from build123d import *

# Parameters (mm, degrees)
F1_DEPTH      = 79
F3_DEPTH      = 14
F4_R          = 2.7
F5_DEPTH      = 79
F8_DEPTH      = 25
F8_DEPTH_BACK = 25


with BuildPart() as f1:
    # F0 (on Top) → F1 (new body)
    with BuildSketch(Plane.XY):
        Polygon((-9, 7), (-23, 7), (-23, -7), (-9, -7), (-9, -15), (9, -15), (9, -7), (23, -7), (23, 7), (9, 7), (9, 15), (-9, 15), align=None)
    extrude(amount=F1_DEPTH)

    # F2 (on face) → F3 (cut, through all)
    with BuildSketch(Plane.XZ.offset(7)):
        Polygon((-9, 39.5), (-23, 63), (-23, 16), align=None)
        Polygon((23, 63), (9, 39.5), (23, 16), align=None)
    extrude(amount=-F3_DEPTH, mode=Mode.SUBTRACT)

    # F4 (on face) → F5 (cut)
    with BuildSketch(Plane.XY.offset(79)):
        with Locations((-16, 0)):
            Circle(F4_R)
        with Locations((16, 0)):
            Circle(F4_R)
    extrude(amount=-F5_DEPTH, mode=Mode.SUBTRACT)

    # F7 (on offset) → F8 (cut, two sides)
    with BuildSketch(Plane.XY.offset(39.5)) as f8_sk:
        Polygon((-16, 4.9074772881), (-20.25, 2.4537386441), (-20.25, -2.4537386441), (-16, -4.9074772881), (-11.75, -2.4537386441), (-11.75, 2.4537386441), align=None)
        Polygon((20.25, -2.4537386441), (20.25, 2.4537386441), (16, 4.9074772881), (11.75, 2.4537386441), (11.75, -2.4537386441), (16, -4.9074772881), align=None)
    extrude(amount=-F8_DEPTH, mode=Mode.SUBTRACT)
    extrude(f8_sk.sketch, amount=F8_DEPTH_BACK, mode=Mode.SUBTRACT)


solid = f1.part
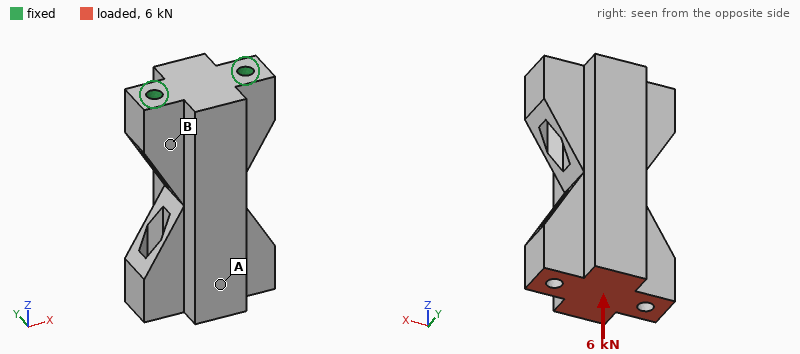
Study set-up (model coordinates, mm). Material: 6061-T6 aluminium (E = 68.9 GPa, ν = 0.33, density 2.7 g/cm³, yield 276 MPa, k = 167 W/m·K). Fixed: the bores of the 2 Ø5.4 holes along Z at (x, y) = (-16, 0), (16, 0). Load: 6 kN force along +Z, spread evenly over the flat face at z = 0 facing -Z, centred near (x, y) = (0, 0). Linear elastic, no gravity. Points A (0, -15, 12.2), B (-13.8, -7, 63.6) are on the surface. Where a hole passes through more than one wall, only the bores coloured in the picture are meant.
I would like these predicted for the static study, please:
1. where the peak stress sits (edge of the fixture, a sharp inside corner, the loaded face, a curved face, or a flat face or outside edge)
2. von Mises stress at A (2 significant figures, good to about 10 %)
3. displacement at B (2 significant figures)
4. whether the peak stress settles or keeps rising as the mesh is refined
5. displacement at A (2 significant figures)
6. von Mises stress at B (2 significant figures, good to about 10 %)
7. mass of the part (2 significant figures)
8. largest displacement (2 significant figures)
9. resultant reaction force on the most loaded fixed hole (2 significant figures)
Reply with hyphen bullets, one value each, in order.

- edge of the fixture
- 7.2 MPa
- 2.5 µm
- keeps rising
- 11 µm
- 16 MPa
- 160 g
- 14 µm
- 3.1 kN
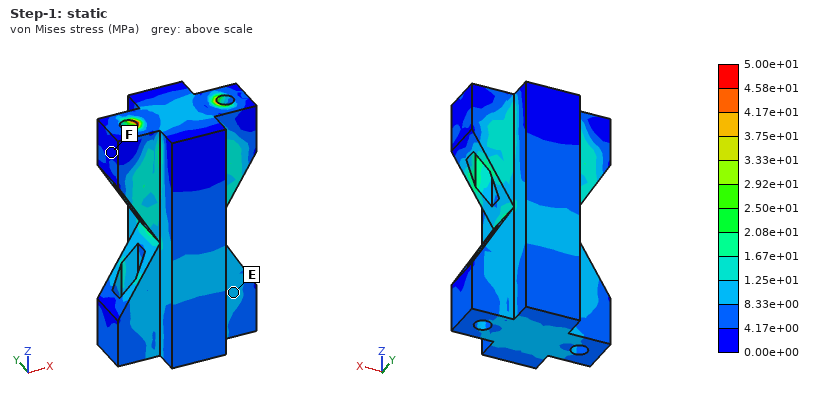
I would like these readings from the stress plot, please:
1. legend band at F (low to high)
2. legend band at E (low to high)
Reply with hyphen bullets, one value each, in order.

- 0.00e+00 to 4.17e+00 MPa
- 8.33e+00 to 1.25e+01 MPa
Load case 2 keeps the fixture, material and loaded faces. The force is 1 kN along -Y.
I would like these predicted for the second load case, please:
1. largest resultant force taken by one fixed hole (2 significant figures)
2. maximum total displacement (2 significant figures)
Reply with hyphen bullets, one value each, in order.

- 500 N
- 0.13 mm
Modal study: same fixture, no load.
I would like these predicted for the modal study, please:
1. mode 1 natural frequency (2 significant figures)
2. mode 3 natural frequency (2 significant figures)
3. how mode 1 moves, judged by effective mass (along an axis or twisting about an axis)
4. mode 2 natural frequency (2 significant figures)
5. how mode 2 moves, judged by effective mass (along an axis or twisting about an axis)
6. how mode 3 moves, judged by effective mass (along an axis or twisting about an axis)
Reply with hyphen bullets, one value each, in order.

- 2000 Hz
- 7400 Hz
- along Y
- 3300 Hz
- along X
- twisting about Z
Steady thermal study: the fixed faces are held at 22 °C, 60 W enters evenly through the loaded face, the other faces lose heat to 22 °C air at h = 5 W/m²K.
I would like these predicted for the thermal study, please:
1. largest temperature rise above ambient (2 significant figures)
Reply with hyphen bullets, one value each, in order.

- 40 K
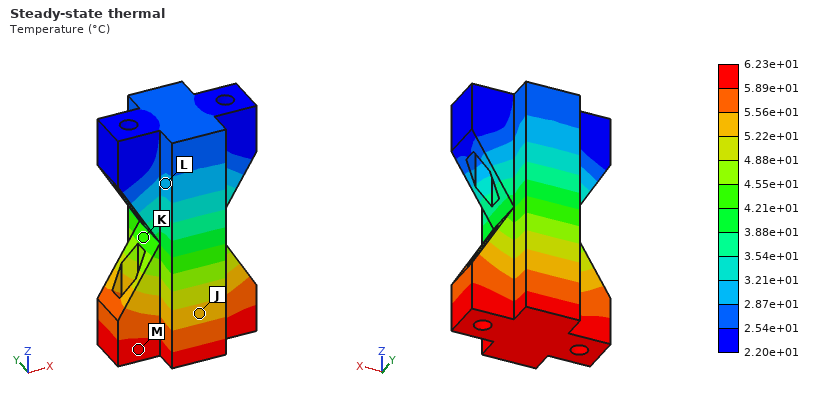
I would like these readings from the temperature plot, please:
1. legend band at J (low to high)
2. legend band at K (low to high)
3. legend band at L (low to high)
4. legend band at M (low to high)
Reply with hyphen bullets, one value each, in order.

- 5.22e+01 to 5.56e+01 °C
- 4.21e+01 to 4.55e+01 °C
- 2.87e+01 to 3.21e+01 °C
- 5.89e+01 to 6.23e+01 °C
